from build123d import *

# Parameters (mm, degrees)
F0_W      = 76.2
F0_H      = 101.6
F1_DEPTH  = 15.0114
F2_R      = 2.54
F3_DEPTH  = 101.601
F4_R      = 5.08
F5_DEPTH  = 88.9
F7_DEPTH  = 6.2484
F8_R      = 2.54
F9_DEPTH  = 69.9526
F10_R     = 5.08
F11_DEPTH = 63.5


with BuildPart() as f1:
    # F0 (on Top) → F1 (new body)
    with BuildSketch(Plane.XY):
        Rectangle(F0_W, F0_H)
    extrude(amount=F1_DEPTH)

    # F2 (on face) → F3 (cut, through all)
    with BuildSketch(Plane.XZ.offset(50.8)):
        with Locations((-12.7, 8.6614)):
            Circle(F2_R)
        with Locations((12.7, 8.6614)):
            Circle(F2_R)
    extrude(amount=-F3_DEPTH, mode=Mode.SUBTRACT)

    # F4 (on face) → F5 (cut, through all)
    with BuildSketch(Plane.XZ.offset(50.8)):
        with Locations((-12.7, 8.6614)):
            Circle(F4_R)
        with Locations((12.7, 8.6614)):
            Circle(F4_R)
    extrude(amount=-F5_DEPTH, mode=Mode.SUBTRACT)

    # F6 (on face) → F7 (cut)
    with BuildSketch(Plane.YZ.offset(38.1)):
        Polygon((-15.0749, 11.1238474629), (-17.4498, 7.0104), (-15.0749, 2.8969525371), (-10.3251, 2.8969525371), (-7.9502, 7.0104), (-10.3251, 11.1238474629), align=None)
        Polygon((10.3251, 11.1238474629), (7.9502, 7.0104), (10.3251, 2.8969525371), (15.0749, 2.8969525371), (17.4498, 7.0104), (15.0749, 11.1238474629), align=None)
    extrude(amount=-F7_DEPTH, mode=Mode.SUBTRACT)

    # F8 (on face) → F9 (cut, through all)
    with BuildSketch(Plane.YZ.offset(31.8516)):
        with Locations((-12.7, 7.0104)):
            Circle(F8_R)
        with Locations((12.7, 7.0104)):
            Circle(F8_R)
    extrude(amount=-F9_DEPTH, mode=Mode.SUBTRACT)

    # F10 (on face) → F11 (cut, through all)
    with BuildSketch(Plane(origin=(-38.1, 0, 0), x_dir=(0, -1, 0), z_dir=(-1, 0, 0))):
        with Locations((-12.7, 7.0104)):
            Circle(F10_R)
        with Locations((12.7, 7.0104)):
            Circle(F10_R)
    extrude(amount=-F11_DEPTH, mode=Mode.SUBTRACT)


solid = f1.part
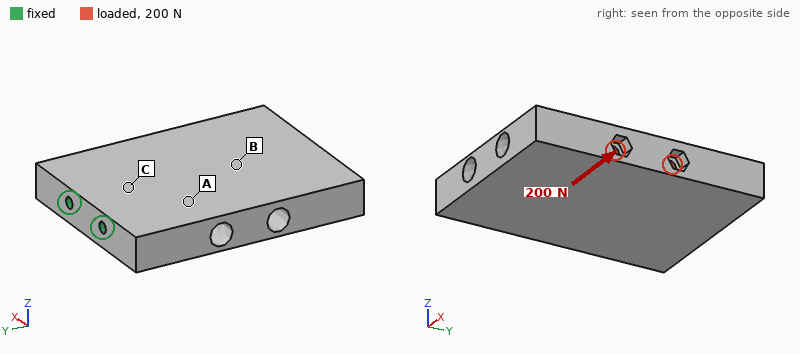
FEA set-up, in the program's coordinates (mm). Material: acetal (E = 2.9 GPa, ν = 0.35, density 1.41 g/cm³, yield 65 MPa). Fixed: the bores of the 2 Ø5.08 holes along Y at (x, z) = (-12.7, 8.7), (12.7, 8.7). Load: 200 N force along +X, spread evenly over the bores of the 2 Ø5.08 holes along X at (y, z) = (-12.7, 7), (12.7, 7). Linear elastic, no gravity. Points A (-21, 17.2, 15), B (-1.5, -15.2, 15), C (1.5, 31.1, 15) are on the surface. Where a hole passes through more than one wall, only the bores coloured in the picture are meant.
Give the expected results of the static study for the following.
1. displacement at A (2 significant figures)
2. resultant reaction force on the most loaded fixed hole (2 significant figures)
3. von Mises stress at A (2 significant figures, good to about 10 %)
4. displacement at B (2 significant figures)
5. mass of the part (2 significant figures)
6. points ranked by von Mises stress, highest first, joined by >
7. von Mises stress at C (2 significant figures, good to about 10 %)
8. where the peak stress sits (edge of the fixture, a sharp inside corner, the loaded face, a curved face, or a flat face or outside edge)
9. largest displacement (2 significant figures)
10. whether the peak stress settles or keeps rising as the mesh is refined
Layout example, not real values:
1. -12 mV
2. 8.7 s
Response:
1. 30 µm
2. 260 N
3. 0.61 MPa
4. 61 µm
5. 130 g
6. C > A > B
7. 1.2 MPa
8. edge of the fixture
9. 97 µm
10. keeps rising
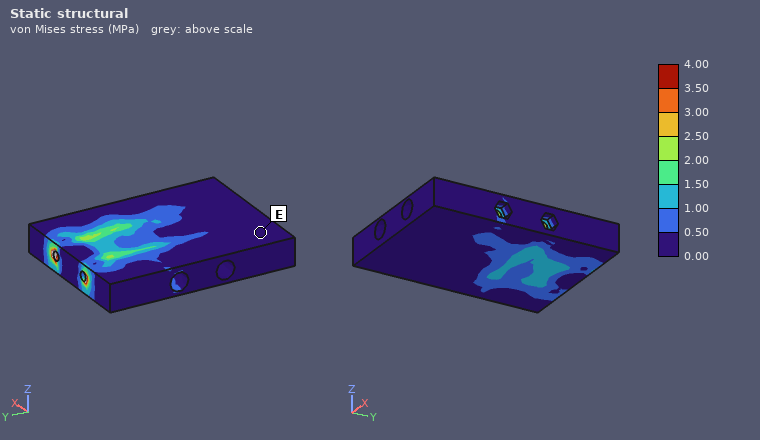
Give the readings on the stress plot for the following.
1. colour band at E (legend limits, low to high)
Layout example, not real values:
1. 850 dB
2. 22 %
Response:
1. 0.00 to 0.50 MPa
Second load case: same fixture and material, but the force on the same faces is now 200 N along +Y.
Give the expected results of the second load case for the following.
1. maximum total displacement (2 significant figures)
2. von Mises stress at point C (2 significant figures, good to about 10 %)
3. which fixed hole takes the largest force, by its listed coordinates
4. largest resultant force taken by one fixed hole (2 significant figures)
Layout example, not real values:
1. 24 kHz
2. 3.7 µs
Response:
1. 63 µm
2. 0.52 MPa
3. (12.7, 8.7)
4. 260 N
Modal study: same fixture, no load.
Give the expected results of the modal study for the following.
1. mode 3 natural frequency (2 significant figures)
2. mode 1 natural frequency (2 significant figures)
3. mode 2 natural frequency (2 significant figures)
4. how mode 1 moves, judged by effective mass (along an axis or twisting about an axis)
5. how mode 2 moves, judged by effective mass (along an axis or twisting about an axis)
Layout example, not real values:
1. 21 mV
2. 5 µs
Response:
1. 780 Hz
2. 310 Hz
3. 720 Hz
4. along Z
5. along X
